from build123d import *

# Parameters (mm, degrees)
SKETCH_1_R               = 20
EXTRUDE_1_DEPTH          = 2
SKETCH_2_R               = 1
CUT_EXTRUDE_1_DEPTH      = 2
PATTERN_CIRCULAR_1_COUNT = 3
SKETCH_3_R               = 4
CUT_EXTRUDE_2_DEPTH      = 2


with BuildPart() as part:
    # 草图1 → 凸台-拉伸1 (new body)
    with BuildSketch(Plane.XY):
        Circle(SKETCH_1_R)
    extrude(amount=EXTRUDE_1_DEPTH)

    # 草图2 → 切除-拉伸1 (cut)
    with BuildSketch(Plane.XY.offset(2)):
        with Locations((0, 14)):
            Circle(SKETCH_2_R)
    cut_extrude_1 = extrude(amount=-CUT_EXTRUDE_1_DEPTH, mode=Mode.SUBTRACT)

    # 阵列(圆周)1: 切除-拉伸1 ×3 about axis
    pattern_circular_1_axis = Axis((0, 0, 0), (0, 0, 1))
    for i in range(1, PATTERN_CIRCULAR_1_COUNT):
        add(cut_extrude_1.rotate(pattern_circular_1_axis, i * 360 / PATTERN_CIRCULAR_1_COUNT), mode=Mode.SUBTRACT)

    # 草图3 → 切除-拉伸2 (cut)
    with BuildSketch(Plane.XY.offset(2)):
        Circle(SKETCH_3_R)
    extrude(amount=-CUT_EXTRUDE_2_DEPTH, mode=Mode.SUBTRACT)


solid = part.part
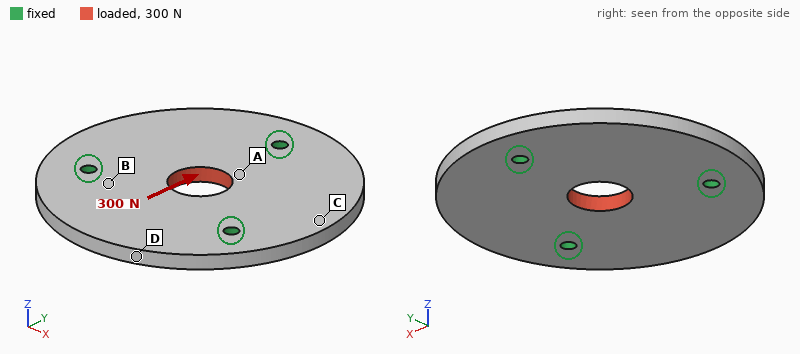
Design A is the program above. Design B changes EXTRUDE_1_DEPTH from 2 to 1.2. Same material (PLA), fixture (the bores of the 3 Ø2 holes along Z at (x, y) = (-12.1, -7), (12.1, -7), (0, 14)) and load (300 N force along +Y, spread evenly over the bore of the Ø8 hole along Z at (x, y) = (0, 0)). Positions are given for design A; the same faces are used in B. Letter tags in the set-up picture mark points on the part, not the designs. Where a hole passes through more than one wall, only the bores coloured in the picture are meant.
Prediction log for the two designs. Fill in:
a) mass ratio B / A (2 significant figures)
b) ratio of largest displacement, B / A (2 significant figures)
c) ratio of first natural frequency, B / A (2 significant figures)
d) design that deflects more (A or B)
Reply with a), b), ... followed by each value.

a) 0.60
b) 1.7
c) 0.64
d) B
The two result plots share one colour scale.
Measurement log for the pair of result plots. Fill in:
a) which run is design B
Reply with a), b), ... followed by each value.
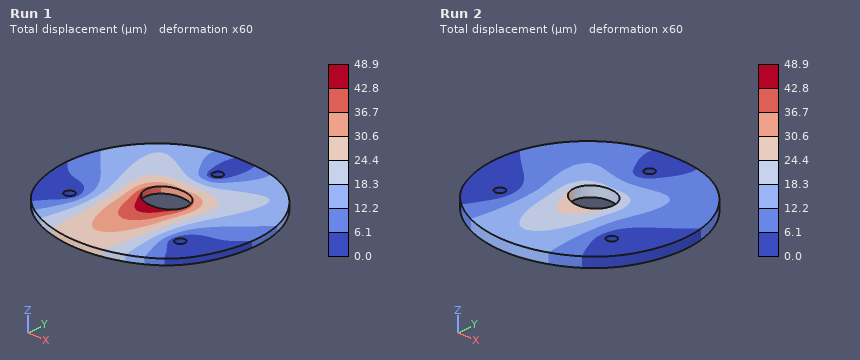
a) Run 1
